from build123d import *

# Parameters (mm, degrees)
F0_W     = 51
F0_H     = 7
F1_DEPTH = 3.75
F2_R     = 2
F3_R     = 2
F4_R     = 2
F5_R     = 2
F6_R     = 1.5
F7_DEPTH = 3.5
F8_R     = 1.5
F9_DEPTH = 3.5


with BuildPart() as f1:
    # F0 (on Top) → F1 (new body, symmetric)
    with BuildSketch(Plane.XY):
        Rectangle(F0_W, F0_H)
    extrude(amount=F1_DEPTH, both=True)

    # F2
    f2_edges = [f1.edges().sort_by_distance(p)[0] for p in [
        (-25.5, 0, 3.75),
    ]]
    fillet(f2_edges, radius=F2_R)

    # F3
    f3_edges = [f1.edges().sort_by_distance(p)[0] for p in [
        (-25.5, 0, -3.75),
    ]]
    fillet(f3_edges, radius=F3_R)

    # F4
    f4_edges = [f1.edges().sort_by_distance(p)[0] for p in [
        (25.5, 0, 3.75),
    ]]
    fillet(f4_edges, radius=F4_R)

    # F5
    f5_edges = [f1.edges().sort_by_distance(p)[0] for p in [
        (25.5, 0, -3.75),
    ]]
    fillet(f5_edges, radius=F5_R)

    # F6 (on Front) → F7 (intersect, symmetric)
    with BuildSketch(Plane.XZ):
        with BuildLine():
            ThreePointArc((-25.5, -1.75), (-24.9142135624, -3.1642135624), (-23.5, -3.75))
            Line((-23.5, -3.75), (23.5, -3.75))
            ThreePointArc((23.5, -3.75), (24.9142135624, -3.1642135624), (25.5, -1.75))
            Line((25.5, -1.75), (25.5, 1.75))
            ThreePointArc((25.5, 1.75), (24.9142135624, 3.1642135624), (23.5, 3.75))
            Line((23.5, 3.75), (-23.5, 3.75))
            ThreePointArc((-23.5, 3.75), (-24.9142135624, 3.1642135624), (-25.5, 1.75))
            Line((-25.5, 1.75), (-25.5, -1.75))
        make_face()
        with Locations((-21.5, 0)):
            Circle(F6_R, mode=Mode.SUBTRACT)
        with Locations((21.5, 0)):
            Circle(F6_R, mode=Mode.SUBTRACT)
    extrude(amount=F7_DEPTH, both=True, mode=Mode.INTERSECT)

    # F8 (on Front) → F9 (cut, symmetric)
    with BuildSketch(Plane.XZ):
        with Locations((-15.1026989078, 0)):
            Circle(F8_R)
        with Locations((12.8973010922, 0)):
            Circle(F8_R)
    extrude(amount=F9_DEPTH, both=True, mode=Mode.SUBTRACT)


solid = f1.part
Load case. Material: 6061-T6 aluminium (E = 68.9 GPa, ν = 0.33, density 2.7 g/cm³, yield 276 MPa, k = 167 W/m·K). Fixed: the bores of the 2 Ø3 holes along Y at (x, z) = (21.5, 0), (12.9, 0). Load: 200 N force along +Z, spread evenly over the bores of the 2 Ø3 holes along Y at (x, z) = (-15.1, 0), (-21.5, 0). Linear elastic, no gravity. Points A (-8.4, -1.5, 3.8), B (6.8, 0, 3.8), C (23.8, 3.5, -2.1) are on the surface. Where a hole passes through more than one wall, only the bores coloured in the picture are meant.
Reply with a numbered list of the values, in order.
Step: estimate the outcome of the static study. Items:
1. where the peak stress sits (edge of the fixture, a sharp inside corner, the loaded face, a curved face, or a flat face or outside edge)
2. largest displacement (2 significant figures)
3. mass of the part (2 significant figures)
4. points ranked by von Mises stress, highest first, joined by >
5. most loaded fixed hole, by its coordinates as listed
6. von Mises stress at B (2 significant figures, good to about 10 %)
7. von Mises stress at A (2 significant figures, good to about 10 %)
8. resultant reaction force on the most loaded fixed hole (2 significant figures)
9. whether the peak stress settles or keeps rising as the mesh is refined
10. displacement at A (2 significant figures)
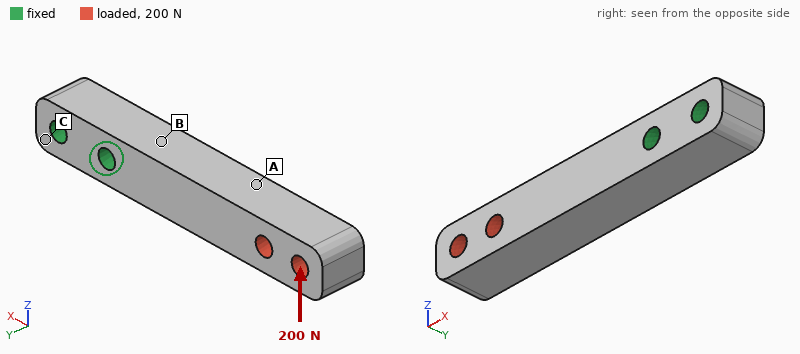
1. edge of the fixture
2. 0.19 mm
3. 6.6 g
4. B > A > C
5. (12.9, 0)
6. 77 MPa
7. 30 MPa
8. 440 N
9. keeps rising
10. 0.081 mm
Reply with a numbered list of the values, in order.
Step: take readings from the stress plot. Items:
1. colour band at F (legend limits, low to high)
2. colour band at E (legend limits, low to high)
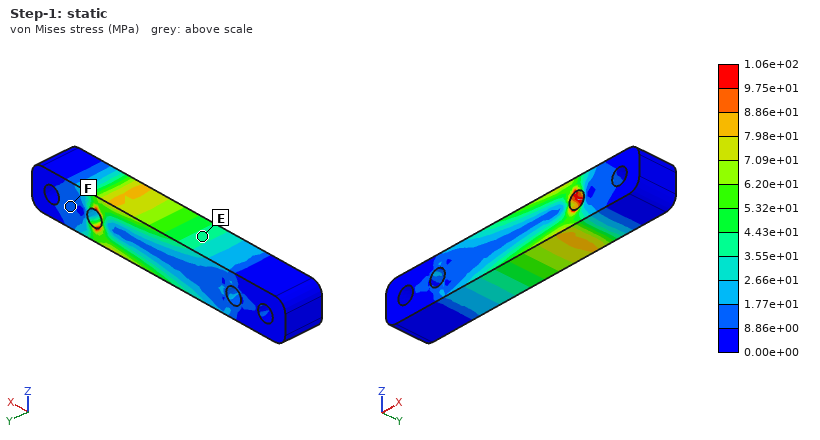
1. 8.86e+00 to 1.77e+01 MPa
2. 3.55e+01 to 4.43e+01 MPa
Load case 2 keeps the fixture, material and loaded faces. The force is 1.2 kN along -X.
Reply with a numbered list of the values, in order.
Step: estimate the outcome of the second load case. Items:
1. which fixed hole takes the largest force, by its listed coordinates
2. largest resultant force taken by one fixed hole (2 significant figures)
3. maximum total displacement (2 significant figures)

1. (12.9, 0)
2. 1.1 kN
3. 12 µm
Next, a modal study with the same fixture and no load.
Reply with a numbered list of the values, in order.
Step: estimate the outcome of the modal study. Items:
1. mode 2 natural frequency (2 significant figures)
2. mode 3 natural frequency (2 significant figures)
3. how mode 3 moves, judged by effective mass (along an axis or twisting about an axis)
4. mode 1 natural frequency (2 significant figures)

1. 4100 Hz
2. 19 kHz
3. twisting about X
4. 4100 Hz
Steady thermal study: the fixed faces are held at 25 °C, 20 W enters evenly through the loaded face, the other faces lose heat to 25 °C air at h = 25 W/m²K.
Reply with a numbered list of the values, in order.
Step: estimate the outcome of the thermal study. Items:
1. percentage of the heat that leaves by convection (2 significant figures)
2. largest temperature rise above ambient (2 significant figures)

1. 5.6 %
2. 72 K
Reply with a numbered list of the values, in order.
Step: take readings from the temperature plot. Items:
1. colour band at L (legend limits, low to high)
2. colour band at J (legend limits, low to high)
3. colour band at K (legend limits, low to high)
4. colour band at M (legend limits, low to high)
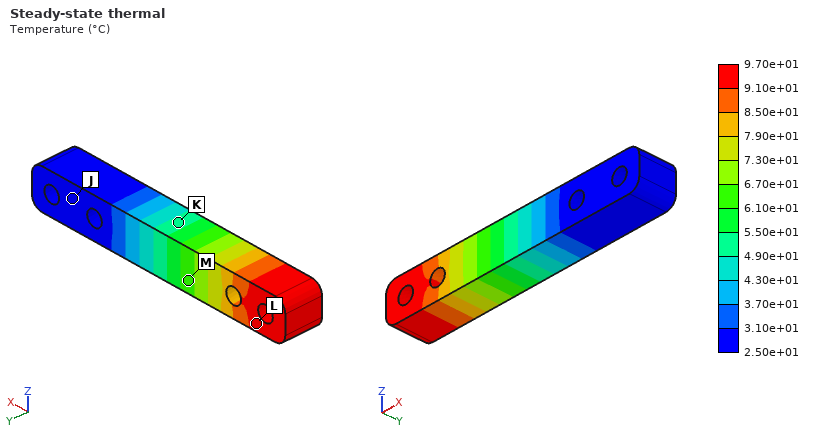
1. 9.10e+01 to 9.70e+01 °C
2. 2.50e+01 to 3.10e+01 °C
3. 4.90e+01 to 5.50e+01 °C
4. 6.10e+01 to 6.70e+01 °C
